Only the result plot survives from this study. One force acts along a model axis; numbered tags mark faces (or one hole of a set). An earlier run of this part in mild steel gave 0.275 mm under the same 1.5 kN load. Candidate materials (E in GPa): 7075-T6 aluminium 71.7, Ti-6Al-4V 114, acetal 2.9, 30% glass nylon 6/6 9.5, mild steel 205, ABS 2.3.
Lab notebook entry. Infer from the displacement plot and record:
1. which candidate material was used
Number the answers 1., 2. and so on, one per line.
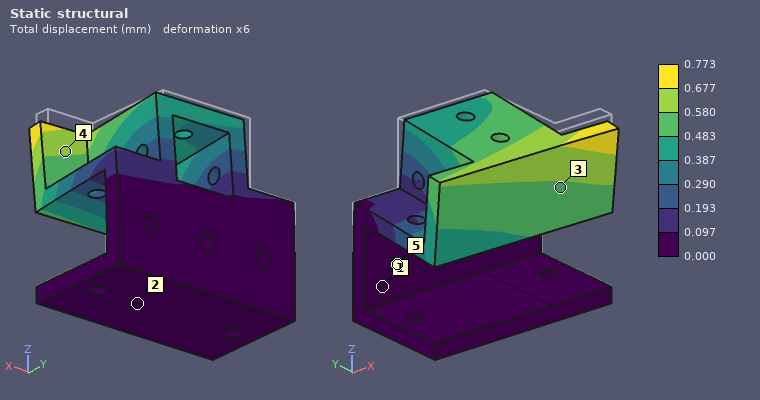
1. 7075-T6 aluminium
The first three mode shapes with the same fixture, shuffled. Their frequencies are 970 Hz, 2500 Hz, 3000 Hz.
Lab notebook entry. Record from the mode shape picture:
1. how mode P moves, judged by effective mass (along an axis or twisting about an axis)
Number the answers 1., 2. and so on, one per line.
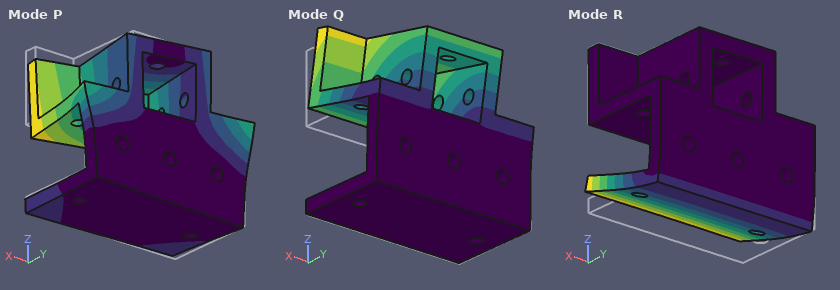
1. along X
